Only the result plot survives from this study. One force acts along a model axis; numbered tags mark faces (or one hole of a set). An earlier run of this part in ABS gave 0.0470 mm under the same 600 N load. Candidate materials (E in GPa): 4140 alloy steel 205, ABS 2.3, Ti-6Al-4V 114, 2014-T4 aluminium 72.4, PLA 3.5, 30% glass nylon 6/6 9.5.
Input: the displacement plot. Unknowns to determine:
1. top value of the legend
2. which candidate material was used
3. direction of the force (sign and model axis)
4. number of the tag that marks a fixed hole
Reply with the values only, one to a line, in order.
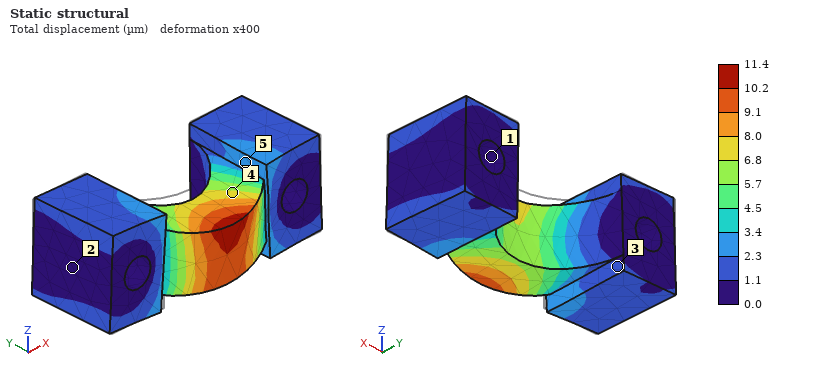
11.4 µm
30% glass nylon 6/6
-Z
1
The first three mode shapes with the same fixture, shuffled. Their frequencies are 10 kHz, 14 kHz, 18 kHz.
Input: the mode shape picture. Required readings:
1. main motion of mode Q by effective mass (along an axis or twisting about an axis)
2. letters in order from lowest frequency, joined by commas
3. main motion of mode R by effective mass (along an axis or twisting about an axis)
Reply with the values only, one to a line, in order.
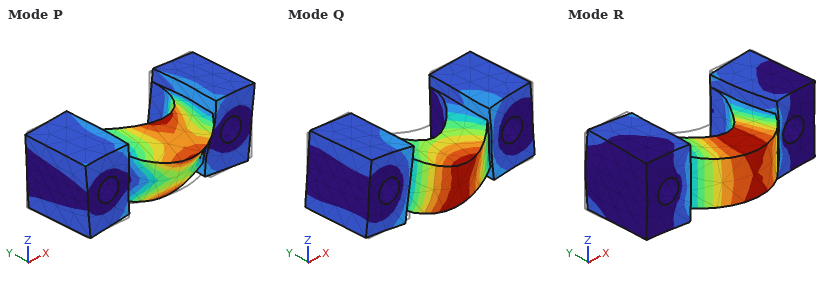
along Z
Q, R, P
along Y
